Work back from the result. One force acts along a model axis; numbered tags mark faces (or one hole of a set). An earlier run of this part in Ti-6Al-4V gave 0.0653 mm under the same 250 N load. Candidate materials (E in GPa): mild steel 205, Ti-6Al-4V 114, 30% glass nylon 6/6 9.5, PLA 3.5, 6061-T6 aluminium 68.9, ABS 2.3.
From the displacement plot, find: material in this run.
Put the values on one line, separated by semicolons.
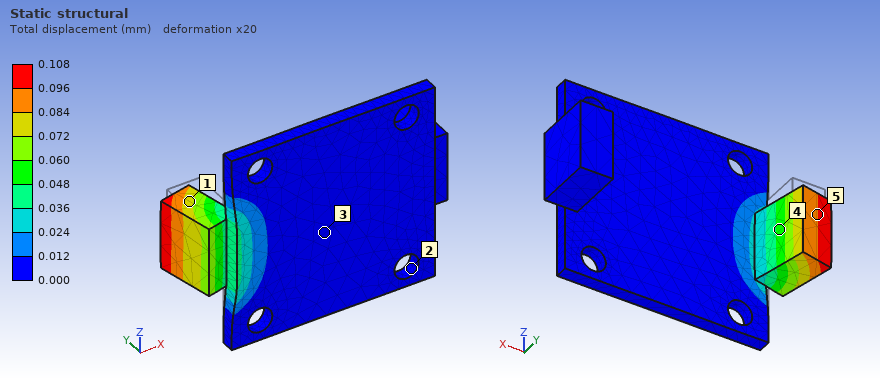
6061-T6 aluminium
